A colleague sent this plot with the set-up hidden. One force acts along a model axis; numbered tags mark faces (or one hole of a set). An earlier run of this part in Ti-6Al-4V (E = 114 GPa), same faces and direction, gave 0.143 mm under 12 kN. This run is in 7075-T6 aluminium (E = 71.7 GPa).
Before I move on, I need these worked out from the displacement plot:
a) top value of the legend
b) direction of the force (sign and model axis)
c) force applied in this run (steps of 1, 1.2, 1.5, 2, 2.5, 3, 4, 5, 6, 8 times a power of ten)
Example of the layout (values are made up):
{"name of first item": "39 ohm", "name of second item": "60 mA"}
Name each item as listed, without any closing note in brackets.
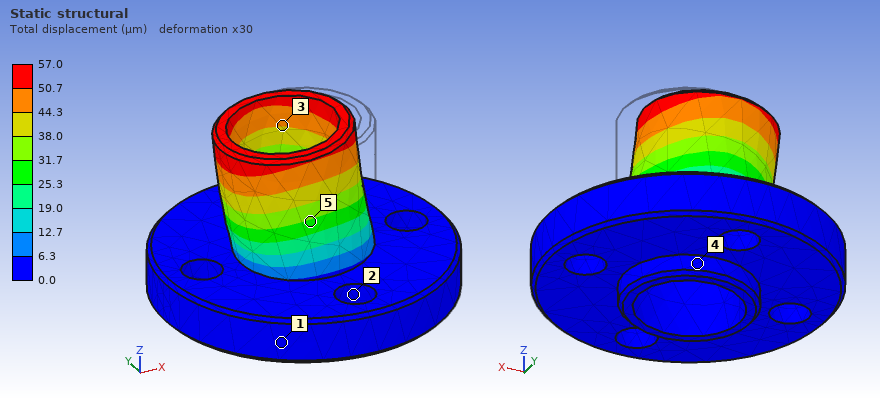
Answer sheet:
{"top value of the legend": "57.0 µm", "direction of the force": "-X", "force applied in this run": "3 kN"}
